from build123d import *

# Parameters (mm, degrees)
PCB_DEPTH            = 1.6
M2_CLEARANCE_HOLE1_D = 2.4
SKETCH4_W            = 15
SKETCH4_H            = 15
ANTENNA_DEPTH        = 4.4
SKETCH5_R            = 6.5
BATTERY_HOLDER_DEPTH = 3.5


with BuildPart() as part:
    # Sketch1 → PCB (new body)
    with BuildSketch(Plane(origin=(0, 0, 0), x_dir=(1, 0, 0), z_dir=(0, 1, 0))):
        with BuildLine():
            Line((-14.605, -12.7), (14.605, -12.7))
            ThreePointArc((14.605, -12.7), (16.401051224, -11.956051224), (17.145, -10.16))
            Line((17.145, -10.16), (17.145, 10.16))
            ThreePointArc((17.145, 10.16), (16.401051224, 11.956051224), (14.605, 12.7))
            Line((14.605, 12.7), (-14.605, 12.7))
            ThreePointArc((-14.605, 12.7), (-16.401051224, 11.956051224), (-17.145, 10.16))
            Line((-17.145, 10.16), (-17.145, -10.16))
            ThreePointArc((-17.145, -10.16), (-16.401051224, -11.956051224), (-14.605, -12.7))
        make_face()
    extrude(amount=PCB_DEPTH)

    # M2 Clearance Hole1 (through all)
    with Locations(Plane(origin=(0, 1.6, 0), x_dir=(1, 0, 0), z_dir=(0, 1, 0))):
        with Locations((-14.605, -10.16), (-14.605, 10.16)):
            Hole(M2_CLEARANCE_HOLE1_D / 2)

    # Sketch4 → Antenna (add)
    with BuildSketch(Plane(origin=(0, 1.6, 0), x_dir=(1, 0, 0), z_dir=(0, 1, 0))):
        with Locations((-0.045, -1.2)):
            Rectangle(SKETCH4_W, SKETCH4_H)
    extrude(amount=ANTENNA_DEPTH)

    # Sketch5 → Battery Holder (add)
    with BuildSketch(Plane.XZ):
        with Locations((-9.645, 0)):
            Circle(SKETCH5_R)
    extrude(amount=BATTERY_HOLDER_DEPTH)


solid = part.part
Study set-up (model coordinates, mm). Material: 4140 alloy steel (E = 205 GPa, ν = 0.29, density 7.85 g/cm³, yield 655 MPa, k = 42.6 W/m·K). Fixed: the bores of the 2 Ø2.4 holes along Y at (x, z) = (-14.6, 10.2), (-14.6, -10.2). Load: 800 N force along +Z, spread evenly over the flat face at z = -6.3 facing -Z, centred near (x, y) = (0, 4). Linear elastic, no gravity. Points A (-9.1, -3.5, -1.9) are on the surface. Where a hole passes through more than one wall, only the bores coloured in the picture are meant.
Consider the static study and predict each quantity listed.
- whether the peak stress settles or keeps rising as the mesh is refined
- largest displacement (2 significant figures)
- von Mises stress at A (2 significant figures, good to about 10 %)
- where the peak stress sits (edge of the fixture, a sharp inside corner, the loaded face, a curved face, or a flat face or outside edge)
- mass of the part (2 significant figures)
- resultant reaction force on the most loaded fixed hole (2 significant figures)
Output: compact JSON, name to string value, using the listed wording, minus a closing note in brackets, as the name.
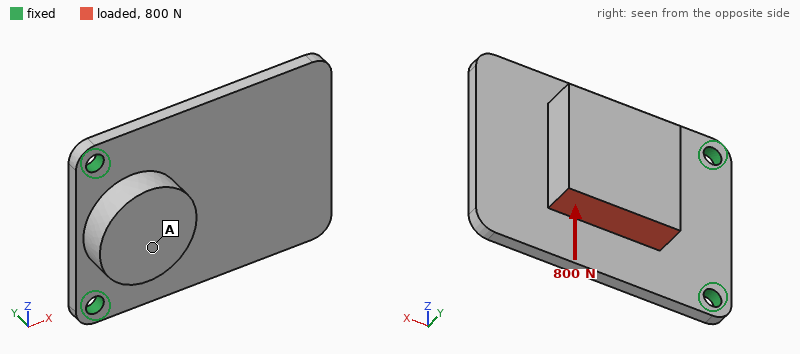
{"whether the peak stress settles or keeps rising as the mesh is refined": "keeps rising", "largest displacement": "16 µm", "von Mises stress at A": "25 MPa", "where the peak stress sits": "edge of the fixture", "mass of the part": "22 g", "resultant reaction force on the most loaded fixed hole": "690 N"}
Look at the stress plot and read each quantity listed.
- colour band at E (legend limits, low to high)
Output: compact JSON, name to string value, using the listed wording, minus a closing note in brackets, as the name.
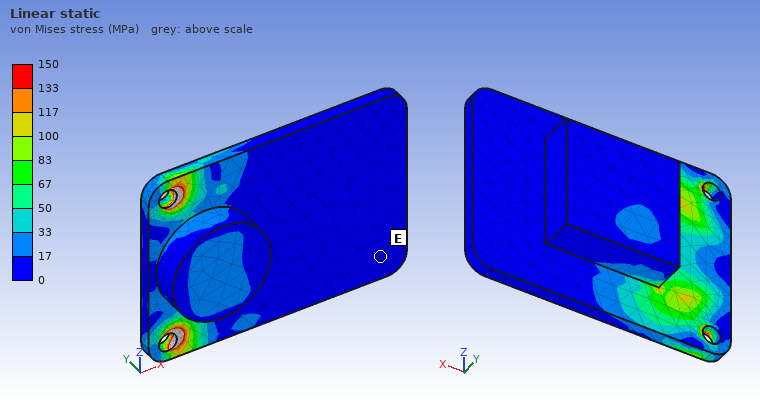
{"colour band at E": "0 to 17 MPa"}
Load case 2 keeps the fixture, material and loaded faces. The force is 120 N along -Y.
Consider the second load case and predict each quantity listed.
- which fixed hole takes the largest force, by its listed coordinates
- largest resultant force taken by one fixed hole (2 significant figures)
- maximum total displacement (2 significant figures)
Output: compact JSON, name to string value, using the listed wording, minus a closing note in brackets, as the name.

{"which fixed hole takes the largest force, by its listed coordinates": "(-14.6, -10.2)", "largest resultant force taken by one fixed hole": "110 N", "maximum total displacement": "0.12 mm"}
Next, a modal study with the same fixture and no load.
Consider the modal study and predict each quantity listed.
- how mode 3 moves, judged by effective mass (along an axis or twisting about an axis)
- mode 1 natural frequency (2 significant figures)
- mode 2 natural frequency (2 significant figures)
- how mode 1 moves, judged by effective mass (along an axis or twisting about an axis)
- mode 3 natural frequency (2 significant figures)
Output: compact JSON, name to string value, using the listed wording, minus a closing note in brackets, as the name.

{"how mode 3 moves, judged by effective mass": "along Y", "mode 1 natural frequency": "1500 Hz", "mode 2 natural frequency": "8800 Hz", "how mode 1 moves, judged by effective mass": "along Y", "mode 3 natural frequency": "11 kHz"}
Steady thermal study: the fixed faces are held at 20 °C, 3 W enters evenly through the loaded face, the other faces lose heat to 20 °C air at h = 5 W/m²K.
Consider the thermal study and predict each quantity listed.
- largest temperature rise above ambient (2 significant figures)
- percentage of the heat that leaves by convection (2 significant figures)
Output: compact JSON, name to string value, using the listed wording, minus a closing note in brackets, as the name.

{"largest temperature rise above ambient": "24 K", "percentage of the heat that leaves by convection": "5.9 %"}
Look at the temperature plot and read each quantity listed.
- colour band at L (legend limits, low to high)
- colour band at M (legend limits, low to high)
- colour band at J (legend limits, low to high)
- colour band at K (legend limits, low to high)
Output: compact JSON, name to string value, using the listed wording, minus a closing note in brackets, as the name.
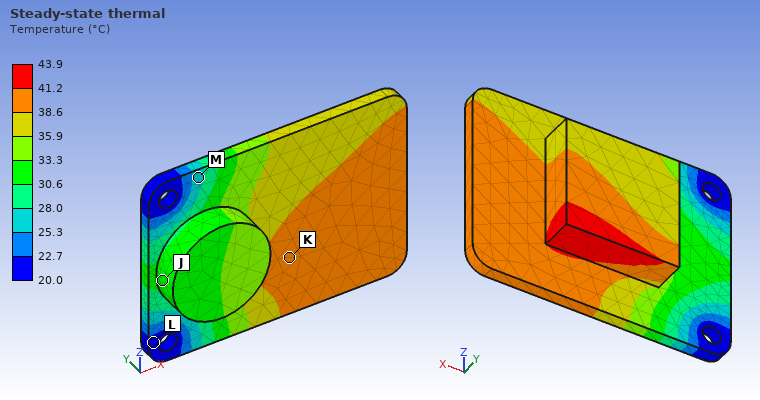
{"colour band at L": "20.0 to 22.7 °C", "colour band at M": "25.3 to 28.0 °C", "colour band at J": "30.6 to 33.3 °C", "colour band at K": "38.6 to 41.2 °C"}
